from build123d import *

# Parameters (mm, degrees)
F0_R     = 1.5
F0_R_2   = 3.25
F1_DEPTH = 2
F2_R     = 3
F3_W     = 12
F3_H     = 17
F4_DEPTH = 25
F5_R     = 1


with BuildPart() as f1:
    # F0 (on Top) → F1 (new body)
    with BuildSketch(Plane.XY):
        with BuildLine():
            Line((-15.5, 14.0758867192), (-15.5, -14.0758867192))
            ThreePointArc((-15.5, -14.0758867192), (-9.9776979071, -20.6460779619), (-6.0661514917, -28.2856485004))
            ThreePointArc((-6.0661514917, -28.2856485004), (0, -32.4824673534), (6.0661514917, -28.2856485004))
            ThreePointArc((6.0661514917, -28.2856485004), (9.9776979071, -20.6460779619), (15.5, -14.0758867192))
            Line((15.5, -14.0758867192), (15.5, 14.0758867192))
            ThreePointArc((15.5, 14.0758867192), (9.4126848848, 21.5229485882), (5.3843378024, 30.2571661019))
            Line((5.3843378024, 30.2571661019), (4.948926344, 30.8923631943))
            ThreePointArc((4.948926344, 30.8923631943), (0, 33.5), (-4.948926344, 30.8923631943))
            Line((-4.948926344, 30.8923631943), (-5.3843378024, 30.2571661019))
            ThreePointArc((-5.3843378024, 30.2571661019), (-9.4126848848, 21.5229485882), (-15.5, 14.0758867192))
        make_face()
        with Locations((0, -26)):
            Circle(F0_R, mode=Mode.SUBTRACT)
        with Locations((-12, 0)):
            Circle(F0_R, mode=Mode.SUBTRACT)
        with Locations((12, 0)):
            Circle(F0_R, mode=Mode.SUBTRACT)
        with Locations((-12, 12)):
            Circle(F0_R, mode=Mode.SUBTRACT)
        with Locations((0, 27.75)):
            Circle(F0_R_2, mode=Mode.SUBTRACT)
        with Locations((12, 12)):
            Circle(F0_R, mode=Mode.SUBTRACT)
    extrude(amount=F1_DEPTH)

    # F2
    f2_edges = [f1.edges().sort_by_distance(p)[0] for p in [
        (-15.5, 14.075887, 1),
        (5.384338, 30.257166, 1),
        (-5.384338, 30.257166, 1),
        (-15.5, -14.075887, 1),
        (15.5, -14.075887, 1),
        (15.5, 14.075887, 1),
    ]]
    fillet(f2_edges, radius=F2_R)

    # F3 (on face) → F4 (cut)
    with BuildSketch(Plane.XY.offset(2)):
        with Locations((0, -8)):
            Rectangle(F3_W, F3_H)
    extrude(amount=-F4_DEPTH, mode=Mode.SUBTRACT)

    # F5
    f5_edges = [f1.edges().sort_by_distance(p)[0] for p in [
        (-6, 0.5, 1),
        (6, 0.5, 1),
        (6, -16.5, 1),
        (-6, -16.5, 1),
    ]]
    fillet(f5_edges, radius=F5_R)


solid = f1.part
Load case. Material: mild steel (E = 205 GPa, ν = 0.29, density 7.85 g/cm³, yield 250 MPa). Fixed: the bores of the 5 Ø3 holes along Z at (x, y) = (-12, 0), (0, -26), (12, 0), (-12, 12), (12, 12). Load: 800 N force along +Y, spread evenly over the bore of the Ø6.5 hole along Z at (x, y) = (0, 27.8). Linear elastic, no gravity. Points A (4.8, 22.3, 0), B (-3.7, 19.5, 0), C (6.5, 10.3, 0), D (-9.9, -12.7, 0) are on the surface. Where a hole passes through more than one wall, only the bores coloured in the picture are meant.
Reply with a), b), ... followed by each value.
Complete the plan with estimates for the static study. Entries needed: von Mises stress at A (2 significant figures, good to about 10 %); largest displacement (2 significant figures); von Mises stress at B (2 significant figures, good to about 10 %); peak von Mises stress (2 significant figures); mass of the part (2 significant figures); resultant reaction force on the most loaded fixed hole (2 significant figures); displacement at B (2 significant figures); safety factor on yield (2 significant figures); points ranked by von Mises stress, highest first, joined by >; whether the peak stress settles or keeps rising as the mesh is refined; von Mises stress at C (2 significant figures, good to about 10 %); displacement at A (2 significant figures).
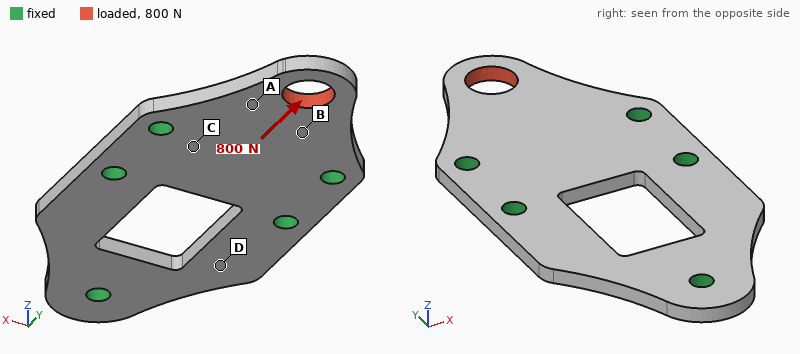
a) 25 MPa
b) 4.1 µm
c) 18 MPa
d) 78 MPa
e) 20 g
f) 310 N
g) 1.3 µm
h) 3.2
i) A > B > C > D
j) settles
k) 13 MPa
l) 1.5 µm
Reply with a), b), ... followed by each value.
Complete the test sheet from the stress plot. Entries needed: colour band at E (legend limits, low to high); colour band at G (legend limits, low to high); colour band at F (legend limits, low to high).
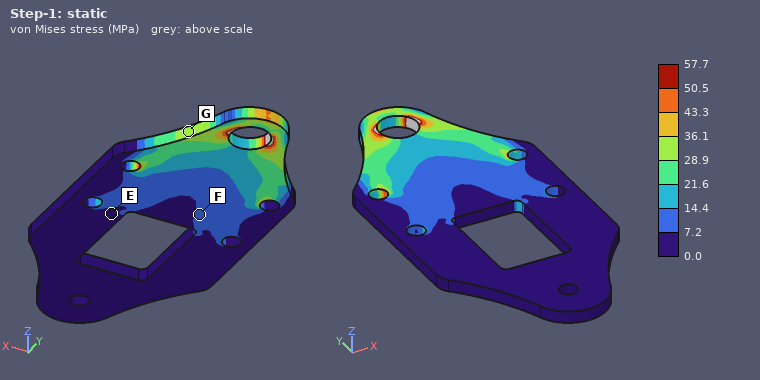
a) 0.0 to 7.2 MPa
b) 28.9 to 36.1 MPa
c) 7.2 to 14.4 MPa
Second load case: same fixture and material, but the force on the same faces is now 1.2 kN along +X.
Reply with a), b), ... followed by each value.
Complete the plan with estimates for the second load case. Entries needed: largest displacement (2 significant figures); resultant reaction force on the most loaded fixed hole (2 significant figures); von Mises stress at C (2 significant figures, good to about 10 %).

a) 19 µm
b) 910 N
c) 13 MPa
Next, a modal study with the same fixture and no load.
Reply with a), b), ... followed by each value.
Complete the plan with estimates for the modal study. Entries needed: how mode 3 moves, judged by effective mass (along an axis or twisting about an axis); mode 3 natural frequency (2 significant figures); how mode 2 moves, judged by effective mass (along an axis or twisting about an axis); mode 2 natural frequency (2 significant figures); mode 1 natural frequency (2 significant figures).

a) along Z
b) 13 kHz
c) twisting about Y
d) 12 kHz
e) 5400 Hz
